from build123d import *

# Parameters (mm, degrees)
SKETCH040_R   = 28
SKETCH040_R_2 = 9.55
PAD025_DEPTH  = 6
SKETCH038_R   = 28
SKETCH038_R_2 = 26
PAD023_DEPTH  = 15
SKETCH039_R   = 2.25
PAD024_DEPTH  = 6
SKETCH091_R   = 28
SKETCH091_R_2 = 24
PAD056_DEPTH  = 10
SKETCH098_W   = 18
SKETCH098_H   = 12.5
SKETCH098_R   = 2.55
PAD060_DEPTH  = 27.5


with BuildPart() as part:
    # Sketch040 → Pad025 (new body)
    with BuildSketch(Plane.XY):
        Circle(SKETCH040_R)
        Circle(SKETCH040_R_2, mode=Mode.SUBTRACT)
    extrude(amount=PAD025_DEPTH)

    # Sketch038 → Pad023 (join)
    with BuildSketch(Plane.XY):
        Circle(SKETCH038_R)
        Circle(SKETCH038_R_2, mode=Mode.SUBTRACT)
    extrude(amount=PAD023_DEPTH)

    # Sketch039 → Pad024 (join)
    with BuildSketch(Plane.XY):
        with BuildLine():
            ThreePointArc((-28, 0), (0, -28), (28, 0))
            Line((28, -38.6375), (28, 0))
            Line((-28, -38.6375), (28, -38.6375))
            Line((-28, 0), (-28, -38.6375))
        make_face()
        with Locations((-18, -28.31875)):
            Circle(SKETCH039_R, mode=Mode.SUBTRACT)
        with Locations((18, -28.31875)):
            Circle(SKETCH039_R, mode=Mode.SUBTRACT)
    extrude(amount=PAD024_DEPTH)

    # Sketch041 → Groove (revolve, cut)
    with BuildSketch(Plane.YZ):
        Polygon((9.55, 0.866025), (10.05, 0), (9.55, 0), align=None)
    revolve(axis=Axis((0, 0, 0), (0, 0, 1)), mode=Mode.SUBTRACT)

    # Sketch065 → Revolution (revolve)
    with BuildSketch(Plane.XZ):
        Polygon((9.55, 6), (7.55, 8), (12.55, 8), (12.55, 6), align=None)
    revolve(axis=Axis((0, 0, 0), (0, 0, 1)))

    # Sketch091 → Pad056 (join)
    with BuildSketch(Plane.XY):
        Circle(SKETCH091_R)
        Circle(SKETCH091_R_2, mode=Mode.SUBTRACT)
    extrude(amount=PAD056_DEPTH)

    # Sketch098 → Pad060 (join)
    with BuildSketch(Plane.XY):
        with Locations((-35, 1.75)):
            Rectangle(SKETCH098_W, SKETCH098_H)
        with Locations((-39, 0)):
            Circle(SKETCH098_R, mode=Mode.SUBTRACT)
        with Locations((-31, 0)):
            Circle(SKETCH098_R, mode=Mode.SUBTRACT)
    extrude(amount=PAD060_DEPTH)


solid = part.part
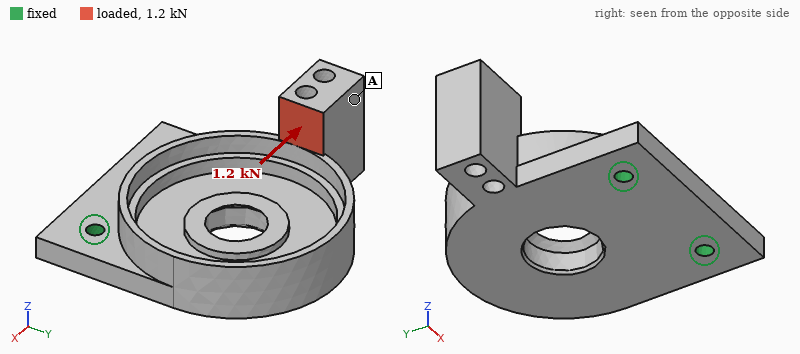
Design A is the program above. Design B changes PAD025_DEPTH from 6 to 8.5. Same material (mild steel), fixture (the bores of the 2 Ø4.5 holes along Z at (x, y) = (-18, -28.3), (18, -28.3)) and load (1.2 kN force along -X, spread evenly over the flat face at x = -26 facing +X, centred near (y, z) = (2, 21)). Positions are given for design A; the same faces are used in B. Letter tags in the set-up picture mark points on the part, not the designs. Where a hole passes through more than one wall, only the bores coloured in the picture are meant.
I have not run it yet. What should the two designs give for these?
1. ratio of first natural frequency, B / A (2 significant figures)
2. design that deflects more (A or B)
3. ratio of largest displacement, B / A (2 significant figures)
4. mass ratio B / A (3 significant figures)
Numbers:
1.0
A
0.64
1.12
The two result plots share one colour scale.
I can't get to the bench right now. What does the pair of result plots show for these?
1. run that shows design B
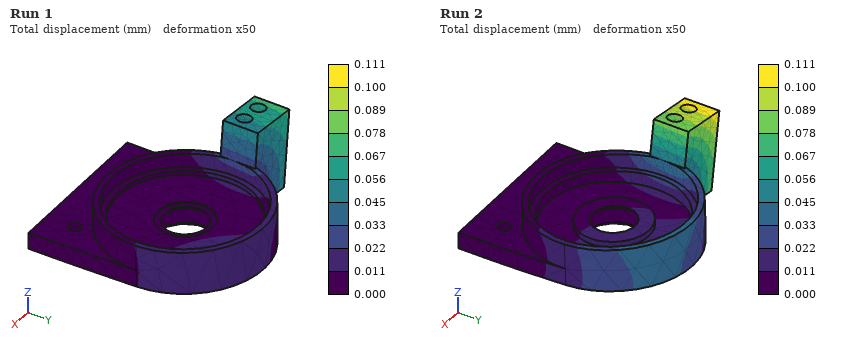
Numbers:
Run 1
